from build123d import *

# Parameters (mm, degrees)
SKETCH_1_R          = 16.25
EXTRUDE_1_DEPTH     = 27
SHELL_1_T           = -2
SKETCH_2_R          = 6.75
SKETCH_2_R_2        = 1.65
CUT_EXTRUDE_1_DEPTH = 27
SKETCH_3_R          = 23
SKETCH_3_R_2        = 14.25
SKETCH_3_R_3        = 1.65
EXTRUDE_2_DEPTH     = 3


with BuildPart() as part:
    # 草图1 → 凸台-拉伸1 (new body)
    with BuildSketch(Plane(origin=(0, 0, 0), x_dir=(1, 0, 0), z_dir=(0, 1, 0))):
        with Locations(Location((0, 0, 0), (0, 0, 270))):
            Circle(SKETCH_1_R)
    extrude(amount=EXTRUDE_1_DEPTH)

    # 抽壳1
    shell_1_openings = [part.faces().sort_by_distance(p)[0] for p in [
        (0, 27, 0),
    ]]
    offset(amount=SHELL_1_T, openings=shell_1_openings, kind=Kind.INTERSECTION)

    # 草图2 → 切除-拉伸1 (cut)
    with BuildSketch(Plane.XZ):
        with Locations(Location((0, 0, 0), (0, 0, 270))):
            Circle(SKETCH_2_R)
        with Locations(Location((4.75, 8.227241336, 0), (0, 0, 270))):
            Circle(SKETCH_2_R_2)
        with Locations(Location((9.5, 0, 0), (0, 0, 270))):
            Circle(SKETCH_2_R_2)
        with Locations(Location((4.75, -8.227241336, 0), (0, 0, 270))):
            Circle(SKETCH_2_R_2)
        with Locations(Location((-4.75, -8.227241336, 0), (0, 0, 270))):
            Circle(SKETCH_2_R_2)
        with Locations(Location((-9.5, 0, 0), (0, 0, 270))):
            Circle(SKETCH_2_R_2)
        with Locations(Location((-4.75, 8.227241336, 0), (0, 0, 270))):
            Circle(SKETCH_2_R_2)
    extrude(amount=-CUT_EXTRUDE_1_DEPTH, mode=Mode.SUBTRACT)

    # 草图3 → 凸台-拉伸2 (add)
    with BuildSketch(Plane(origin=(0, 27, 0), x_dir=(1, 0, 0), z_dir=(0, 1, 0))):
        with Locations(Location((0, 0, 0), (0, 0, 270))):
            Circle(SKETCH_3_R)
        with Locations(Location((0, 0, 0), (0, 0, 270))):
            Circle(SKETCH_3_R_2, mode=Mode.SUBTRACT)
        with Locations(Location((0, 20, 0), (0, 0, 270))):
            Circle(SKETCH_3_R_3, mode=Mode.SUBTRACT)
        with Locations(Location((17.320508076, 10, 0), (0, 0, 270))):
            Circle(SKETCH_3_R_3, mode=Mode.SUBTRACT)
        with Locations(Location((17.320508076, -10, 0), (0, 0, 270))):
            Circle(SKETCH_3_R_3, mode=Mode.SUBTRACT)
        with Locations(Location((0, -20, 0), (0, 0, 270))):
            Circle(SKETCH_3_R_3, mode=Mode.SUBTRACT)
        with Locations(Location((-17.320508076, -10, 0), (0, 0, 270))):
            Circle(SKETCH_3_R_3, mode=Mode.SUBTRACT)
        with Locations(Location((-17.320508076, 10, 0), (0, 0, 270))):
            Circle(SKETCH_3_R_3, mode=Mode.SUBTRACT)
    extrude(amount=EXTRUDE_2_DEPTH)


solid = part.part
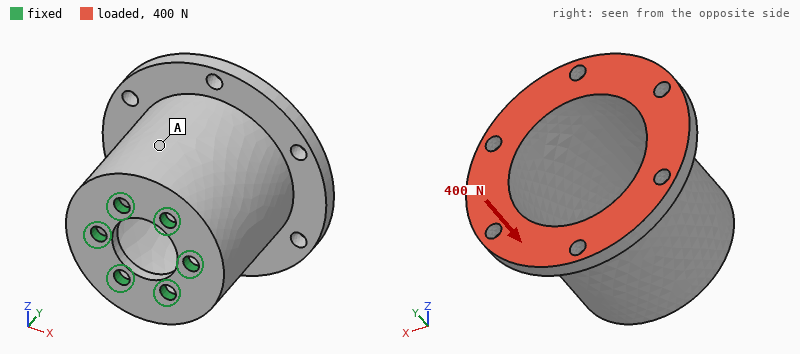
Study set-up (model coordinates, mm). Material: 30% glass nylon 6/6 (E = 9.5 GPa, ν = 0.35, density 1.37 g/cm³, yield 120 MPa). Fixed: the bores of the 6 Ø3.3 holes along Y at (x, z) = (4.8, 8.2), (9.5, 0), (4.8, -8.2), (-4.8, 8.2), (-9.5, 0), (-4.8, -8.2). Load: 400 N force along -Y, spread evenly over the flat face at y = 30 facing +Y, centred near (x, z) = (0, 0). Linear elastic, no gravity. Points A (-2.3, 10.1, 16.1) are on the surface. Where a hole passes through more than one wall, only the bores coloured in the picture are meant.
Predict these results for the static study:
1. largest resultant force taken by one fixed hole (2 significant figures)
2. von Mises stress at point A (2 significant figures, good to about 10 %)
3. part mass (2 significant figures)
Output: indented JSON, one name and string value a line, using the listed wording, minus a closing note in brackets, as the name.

{
  "largest resultant force taken by one fixed hole": "69 N",
  "von Mises stress at point A": "2.6 MPa",
  "part mass": "12 g"
}
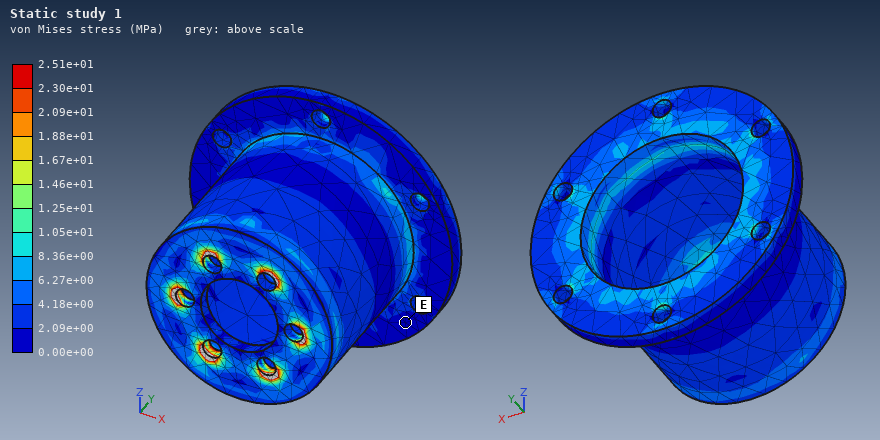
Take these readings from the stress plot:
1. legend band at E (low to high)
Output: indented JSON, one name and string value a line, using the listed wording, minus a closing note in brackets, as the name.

{
  "legend band at E": "0.00e+00 to 2.09e+00 MPa"
}
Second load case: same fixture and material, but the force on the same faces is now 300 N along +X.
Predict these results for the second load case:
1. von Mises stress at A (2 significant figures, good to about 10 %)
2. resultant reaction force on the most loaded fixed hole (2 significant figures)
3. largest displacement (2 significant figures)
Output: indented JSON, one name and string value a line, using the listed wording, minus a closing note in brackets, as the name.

{
  "von Mises stress at A": "6.5 MPa",
  "resultant reaction force on the most loaded fixed hole": "210 N",
  "largest displacement": "0.23 mm"
}
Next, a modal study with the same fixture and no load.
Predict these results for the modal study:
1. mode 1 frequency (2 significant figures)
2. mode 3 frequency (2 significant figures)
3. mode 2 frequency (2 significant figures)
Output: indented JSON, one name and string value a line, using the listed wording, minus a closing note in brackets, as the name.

{
  "mode 1 frequency": "2500 Hz",
  "mode 3 frequency": "6200 Hz",
  "mode 2 frequency": "2500 Hz"
}
